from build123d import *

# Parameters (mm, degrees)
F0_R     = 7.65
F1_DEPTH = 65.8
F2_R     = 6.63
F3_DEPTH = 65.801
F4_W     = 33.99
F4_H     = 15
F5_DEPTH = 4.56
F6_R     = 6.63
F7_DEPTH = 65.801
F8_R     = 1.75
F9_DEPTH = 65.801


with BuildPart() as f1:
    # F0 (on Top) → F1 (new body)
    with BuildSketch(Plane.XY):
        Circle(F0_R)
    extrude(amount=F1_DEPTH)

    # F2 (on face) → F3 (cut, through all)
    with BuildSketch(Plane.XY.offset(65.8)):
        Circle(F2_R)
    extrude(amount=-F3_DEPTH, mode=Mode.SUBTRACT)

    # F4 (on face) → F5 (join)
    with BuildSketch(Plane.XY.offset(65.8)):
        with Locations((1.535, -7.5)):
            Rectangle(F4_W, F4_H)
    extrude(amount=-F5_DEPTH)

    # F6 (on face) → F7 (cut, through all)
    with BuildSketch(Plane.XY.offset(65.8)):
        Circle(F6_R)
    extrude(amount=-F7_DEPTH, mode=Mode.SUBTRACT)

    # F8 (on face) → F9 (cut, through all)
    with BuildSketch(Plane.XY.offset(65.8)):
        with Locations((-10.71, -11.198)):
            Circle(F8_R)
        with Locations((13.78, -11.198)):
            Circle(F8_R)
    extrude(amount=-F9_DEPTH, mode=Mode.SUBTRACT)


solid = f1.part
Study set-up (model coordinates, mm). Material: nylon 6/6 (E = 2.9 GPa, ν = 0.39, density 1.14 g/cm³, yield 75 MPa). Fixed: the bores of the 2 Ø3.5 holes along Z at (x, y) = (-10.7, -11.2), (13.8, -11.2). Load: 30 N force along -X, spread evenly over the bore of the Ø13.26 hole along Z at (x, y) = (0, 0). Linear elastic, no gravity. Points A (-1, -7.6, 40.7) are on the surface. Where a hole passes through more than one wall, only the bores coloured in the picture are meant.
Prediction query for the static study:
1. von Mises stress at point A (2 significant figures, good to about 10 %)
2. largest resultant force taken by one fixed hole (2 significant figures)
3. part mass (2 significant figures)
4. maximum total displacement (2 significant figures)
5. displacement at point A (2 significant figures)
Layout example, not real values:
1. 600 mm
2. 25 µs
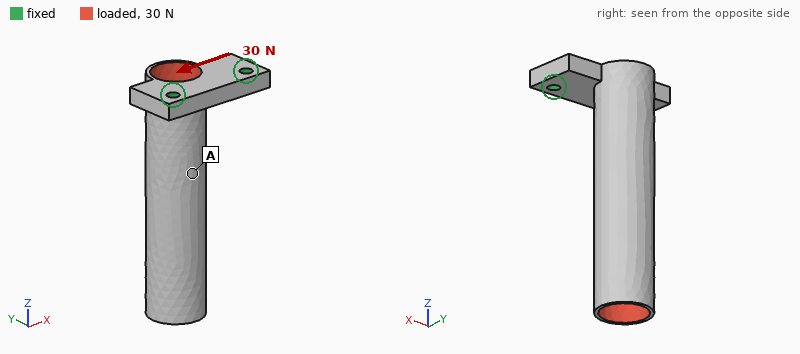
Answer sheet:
1. 1.3 MPa
2. 52 N
3. 5.5 g
4. 0.80 mm
5. 0.24 mm
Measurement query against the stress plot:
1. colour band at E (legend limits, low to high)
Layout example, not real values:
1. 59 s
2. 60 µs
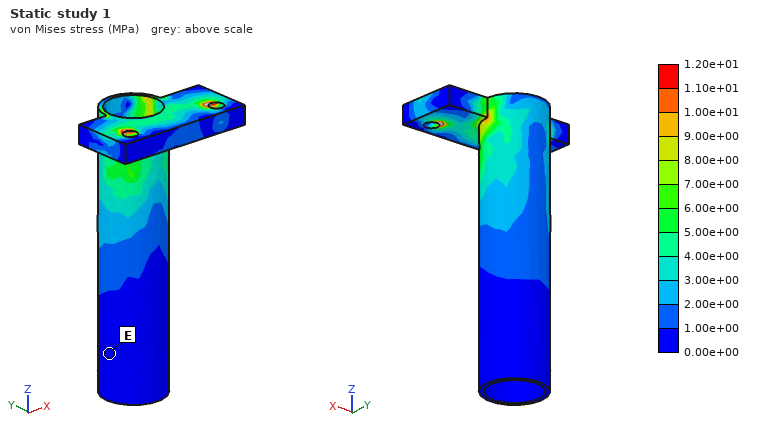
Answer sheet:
1. 0.00e+00 to 1.00e+00 MPa
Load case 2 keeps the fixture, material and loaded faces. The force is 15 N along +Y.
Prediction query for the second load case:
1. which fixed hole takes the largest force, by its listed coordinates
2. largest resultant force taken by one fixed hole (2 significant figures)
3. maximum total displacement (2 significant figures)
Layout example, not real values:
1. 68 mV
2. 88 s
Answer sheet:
1. (-10.7, -11.2)
2. 10 N
3. 0.88 mm
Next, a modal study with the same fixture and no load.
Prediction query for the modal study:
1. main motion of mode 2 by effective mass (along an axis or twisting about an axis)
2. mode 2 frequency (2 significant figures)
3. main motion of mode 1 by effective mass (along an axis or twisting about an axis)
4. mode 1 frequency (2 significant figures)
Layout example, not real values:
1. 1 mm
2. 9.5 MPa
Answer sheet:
1. along X
2. 640 Hz
3. along Y
4. 430 Hz
